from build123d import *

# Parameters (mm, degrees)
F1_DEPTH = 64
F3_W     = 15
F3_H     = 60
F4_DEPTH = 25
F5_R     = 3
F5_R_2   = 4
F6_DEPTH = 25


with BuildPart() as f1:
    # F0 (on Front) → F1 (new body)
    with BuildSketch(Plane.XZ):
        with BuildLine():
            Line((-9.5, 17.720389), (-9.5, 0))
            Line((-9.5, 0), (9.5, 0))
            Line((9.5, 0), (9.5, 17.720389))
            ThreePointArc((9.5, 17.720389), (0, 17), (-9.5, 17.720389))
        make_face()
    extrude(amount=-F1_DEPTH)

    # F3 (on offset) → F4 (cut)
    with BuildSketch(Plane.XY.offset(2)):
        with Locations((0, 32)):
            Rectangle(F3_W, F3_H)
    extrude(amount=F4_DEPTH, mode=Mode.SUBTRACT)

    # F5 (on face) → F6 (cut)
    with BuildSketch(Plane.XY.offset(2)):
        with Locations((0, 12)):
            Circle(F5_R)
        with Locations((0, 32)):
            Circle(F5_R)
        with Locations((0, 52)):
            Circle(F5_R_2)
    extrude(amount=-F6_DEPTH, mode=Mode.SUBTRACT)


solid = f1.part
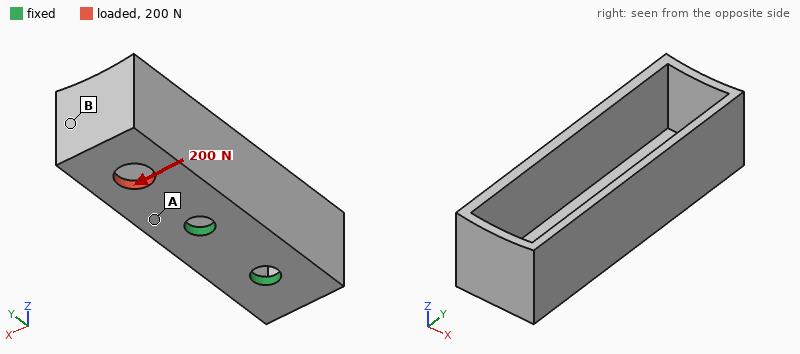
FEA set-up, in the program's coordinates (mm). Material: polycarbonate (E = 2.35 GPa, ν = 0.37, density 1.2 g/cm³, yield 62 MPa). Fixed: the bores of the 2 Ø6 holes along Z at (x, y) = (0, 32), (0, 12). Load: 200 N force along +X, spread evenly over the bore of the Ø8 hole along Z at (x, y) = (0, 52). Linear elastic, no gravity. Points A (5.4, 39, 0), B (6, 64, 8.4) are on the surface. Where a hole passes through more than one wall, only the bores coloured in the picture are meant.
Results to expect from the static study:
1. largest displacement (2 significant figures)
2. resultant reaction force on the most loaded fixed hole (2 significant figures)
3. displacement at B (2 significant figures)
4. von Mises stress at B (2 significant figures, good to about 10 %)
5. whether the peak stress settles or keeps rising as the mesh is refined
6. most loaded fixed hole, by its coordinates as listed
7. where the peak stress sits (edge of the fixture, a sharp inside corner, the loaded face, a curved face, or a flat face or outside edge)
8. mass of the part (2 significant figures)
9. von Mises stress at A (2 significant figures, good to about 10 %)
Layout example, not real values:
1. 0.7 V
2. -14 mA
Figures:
1. 0.78 mm
2. 310 N
3. 0.65 mm
4. 2.8 MPa
5. keeps rising
6. (0, 32)
7. edge of the fixture
8. 8.5 g
9. 9.4 MPa
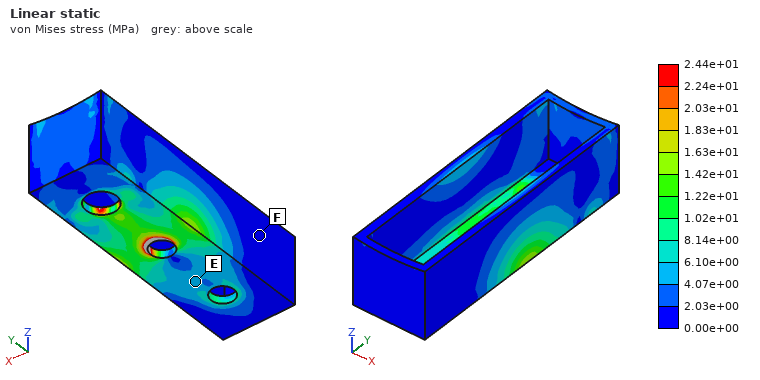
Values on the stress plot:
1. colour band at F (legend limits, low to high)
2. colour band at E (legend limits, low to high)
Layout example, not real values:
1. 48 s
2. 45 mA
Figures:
1. 0.00e+00 to 2.03e+00 MPa
2. 4.07e+00 to 6.10e+00 MPa
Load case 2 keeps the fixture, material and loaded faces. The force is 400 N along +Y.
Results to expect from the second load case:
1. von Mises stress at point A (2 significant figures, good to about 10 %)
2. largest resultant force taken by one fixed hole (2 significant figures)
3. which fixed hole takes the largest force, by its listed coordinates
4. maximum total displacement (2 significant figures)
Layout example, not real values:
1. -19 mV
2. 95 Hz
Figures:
1. 9.0 MPa
2. 330 N
3. (0, 32)
4. 0.17 mm
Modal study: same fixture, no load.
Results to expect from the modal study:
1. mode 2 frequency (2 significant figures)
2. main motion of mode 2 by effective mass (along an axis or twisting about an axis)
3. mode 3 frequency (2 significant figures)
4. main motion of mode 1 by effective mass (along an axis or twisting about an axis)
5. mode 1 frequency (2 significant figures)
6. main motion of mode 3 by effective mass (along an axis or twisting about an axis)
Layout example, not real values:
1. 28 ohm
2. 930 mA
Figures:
1. 1000 Hz
2. along Z
3. 1300 Hz
4. along X
5. 770 Hz
6. along X
